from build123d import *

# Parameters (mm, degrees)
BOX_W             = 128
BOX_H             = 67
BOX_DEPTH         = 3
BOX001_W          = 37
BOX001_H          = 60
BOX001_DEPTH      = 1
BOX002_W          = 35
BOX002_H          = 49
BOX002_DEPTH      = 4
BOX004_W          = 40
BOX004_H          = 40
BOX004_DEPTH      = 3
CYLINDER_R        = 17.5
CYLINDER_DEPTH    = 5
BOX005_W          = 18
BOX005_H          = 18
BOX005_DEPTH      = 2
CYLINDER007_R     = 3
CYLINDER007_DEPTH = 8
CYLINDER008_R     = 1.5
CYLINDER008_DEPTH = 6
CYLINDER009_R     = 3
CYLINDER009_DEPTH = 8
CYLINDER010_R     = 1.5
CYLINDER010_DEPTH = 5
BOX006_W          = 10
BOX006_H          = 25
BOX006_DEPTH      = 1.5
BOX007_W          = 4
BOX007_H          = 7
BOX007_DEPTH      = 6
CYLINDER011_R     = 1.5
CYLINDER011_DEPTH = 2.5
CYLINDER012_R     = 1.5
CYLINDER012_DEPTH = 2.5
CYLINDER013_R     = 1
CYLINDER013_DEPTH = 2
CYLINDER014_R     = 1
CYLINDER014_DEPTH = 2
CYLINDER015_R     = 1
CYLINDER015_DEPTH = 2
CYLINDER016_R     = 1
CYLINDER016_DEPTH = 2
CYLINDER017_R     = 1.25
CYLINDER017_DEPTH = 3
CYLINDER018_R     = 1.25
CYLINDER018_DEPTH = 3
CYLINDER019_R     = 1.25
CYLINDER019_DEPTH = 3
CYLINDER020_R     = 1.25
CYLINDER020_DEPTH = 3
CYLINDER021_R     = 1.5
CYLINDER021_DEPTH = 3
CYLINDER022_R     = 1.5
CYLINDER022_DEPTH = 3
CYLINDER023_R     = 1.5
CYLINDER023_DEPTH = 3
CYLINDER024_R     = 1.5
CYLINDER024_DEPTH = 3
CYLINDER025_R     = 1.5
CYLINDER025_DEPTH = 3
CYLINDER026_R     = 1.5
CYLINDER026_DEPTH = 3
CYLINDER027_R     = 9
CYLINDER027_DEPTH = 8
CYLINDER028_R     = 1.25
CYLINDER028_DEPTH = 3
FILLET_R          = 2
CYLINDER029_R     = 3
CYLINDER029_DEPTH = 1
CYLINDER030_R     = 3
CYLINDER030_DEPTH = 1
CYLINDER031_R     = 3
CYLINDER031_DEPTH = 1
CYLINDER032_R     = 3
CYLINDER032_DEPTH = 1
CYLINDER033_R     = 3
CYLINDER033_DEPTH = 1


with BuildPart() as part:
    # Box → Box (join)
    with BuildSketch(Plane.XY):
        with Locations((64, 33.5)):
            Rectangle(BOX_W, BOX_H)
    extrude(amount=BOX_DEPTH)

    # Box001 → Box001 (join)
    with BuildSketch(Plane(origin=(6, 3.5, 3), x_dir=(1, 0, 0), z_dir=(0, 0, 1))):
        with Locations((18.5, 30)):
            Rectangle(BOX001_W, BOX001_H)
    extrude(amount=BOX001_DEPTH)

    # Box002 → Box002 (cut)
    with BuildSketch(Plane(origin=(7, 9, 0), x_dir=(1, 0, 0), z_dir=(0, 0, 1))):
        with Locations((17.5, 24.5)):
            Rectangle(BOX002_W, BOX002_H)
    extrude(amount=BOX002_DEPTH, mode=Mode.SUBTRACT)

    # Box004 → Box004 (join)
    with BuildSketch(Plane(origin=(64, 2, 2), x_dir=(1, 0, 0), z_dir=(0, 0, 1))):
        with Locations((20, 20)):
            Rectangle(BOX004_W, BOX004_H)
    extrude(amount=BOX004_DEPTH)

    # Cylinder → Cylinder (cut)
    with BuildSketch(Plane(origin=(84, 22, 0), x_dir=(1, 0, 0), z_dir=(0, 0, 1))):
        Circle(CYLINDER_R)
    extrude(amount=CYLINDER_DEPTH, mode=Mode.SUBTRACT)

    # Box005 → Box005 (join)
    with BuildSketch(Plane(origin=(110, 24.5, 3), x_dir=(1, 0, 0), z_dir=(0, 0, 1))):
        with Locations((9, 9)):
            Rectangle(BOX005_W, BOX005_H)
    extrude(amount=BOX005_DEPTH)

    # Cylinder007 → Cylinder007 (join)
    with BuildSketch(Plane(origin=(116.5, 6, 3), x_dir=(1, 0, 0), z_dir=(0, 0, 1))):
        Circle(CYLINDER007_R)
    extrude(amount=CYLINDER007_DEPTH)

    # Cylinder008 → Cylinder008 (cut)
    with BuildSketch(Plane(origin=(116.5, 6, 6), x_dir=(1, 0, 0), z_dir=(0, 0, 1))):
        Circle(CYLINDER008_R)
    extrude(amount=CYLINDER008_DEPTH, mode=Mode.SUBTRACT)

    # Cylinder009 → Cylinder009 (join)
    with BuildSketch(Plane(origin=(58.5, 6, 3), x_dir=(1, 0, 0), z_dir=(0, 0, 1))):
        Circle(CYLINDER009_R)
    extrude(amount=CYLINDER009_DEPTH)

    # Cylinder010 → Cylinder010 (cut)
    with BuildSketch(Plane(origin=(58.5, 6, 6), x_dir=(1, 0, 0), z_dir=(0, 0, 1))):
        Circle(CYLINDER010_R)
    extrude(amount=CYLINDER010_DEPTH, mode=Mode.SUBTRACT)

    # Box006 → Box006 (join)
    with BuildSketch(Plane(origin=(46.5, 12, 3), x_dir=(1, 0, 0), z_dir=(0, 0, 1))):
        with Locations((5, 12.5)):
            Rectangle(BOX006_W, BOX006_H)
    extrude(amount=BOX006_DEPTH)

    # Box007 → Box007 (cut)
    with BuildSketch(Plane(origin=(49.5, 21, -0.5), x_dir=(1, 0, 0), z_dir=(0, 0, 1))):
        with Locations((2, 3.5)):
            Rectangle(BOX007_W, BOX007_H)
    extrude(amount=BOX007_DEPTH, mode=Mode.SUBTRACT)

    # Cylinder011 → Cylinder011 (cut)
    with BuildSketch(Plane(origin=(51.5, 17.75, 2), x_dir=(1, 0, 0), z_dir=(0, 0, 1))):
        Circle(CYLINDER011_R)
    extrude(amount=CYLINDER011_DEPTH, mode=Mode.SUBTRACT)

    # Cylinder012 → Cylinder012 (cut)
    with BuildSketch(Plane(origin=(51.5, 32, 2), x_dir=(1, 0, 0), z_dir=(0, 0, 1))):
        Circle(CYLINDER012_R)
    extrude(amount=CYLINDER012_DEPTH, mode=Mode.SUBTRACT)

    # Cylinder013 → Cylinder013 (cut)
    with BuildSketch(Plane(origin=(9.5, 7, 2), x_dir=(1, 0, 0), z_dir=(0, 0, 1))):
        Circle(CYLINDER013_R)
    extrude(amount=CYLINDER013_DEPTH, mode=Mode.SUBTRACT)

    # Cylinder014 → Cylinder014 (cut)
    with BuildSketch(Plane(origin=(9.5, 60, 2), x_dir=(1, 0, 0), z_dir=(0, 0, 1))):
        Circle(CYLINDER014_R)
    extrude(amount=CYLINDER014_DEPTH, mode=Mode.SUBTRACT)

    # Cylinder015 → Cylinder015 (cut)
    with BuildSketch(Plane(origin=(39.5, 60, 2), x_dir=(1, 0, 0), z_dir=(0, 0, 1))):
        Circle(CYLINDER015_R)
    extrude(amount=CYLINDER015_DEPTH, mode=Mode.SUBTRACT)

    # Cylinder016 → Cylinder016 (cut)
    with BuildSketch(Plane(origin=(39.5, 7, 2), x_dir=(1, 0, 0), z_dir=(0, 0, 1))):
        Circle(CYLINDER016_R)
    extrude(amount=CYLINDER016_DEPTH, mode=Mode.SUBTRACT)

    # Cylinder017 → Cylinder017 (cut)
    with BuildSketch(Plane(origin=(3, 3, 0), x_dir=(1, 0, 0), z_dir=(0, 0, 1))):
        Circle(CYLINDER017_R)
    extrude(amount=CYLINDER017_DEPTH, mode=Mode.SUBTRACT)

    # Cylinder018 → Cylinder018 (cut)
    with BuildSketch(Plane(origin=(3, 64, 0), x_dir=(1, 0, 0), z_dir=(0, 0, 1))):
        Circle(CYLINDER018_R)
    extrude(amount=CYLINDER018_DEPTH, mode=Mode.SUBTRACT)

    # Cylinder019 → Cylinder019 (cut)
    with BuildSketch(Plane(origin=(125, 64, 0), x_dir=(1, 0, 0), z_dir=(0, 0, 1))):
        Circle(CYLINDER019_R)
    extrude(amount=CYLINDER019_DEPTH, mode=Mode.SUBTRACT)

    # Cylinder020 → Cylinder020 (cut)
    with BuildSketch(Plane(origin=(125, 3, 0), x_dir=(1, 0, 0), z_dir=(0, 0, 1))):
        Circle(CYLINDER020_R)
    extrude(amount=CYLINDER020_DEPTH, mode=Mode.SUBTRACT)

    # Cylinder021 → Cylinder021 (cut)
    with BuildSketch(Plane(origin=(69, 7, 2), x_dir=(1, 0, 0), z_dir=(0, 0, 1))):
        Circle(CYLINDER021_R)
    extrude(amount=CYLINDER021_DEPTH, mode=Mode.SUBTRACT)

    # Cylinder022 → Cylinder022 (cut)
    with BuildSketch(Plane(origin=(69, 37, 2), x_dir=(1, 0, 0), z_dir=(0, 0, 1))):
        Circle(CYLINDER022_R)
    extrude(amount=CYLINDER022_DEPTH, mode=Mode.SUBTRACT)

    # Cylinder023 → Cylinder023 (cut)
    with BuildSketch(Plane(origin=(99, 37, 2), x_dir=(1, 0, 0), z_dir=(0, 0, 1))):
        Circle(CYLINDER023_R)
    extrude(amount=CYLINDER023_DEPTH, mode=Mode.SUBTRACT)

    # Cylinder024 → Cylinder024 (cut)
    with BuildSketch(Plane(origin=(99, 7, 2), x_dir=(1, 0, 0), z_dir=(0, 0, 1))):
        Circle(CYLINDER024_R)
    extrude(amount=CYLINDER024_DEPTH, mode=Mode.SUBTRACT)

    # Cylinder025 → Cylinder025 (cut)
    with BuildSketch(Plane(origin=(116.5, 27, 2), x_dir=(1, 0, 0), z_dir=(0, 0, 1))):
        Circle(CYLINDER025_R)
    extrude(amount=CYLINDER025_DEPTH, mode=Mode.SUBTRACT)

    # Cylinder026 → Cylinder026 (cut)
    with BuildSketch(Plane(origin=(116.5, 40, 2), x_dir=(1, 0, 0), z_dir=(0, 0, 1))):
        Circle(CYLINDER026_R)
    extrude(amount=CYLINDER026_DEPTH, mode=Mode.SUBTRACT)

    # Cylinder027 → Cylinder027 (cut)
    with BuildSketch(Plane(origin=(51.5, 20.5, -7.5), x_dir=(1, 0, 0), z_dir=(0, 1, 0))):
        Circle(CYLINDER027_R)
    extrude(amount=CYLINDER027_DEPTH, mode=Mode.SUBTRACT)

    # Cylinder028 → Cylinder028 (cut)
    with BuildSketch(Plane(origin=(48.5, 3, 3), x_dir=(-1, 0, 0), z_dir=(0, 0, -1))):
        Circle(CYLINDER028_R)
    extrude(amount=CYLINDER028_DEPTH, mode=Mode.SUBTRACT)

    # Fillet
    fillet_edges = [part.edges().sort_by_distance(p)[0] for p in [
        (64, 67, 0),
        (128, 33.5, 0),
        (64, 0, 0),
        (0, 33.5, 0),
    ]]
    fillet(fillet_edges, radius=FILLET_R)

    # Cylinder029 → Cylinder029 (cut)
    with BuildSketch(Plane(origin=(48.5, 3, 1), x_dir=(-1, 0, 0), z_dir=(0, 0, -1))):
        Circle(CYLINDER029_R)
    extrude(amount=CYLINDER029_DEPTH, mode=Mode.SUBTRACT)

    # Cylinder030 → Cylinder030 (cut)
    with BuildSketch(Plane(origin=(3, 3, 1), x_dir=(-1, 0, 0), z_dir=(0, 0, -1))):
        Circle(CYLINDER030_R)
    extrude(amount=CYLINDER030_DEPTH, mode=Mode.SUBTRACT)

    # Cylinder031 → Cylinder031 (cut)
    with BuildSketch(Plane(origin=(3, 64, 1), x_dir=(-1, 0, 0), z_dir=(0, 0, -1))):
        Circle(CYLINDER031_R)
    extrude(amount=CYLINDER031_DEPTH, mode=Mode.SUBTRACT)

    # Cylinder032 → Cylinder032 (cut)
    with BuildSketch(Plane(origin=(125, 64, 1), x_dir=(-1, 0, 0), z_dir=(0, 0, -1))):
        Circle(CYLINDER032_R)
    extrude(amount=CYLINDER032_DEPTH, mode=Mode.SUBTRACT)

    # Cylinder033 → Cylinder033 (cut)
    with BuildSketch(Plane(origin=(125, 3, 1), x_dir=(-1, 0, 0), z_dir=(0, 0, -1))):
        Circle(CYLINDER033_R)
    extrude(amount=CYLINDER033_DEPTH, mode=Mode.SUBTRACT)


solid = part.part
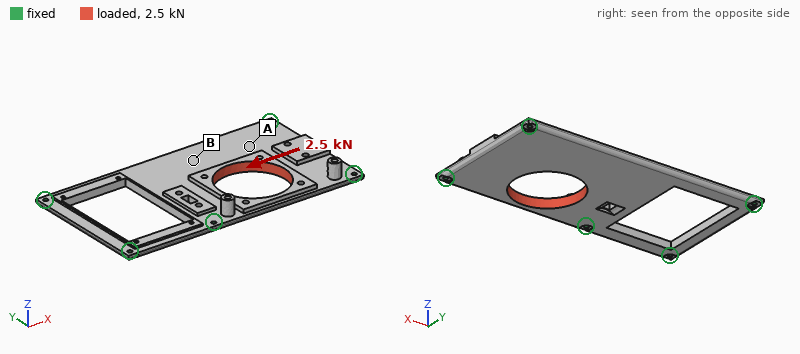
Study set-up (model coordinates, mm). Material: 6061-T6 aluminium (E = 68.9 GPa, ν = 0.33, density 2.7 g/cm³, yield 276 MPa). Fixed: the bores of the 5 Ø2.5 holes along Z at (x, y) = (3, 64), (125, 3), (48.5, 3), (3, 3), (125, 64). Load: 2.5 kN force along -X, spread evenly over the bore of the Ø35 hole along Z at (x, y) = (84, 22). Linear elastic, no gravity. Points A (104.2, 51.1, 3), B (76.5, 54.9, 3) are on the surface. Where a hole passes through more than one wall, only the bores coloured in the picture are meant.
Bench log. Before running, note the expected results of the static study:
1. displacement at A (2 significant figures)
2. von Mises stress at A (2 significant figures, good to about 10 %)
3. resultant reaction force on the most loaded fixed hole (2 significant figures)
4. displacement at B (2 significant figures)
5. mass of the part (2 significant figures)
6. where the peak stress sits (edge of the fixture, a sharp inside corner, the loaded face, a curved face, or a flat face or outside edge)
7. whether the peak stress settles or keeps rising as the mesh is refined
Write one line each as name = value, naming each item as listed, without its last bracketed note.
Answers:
displacement at A = 12 µm
von Mises stress at A = 12 MPa
resultant reaction force on the most loaded fixed hole = 790 N
displacement at B = 13 µm
mass of the part = 54 g
where the peak stress sits = edge of the fixture
whether the peak stress settles or keeps rising as the mesh is refined = keeps rising
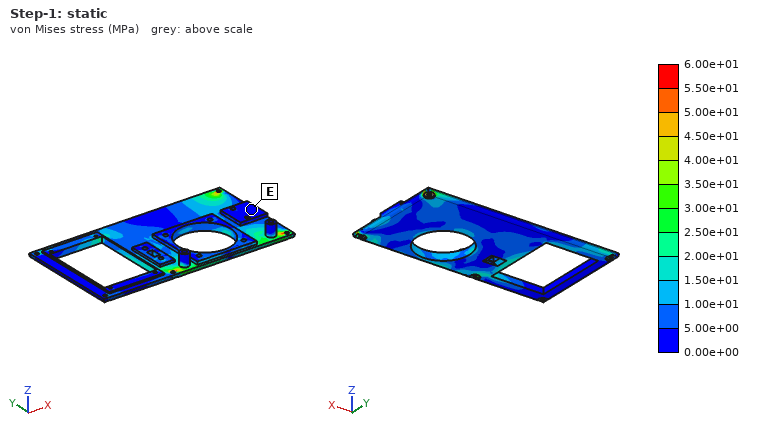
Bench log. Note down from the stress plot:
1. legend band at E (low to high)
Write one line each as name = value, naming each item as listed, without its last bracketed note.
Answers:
legend band at E = 0.00e+00 to 5.00e+00 MPa
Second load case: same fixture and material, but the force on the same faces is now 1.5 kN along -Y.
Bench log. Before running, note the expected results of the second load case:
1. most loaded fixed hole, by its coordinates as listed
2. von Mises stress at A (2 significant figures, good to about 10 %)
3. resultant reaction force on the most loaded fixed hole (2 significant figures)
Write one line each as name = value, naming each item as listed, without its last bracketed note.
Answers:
most loaded fixed hole, by its coordinates as listed = (48.5, 3)
von Mises stress at A = 7.9 MPa
resultant reaction force on the most loaded fixed hole = 710 N
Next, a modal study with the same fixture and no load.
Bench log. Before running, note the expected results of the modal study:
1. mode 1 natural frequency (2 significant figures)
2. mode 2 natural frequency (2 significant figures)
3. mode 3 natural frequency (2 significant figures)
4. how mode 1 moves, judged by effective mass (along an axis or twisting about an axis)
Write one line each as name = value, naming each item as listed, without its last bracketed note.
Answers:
mode 1 natural frequency = 1000 Hz
mode 2 natural frequency = 2300 Hz
mode 3 natural frequency = 3200 Hz
how mode 1 moves, judged by effective mass = along Z
